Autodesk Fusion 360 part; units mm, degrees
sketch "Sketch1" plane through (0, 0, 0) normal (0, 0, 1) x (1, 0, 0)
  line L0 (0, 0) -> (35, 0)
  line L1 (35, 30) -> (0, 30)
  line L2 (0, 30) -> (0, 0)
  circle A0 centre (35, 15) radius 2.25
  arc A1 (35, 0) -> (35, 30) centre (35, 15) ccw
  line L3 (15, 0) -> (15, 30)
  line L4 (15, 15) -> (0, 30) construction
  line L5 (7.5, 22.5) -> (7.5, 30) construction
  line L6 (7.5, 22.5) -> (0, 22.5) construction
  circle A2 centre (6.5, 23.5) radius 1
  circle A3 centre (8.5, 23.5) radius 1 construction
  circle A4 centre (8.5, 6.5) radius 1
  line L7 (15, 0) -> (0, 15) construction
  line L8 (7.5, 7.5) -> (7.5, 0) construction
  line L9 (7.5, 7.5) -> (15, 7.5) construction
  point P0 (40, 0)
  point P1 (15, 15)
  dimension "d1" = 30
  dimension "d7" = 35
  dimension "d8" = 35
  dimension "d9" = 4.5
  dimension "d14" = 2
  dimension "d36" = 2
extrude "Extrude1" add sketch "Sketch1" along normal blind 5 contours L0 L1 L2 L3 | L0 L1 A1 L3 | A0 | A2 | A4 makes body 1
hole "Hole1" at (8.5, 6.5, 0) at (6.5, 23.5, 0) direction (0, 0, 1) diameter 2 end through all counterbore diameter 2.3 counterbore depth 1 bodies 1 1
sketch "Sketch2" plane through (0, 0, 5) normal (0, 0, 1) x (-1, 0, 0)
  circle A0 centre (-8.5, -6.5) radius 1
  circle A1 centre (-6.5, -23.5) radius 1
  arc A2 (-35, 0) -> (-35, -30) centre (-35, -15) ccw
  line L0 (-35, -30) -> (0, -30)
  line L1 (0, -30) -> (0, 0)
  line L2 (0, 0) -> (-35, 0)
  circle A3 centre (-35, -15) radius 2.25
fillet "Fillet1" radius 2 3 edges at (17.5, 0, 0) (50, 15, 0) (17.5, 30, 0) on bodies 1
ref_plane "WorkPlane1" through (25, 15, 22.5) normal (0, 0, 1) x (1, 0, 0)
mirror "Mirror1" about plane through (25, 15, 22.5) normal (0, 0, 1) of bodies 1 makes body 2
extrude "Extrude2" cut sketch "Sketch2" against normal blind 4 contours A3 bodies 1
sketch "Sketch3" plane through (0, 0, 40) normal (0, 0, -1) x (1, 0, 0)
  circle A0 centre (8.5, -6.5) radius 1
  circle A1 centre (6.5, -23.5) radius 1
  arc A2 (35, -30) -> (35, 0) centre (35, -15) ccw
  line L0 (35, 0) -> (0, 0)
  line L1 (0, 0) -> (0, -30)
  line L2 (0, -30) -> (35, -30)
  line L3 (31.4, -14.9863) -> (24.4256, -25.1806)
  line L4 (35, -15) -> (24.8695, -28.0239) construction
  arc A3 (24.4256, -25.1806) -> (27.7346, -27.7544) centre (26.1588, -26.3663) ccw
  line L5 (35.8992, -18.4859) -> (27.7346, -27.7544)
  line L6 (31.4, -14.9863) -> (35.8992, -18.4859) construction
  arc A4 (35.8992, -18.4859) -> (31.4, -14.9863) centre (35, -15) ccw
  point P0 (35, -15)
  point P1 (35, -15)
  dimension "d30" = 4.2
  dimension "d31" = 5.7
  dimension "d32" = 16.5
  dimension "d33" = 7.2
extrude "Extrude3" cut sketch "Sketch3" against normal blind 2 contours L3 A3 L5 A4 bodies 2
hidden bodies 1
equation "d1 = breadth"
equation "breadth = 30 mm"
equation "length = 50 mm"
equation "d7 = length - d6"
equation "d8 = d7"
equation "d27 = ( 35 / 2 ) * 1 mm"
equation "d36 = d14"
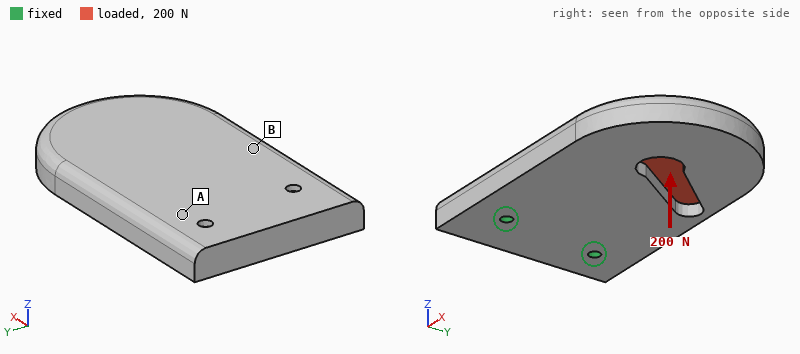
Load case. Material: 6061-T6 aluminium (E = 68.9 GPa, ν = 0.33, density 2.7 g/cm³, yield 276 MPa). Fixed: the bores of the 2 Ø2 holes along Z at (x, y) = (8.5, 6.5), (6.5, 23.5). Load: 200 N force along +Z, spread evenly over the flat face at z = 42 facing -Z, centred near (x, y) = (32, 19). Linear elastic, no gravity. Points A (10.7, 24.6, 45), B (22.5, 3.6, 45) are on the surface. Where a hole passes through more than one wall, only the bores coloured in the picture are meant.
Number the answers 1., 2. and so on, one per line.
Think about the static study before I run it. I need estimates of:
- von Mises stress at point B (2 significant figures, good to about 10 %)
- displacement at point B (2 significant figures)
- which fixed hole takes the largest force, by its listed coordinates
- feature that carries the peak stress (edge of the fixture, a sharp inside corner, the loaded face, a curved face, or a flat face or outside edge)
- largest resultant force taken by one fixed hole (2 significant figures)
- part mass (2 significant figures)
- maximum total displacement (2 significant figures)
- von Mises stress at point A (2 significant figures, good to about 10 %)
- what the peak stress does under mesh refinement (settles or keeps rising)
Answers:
1. 17 MPa
2. 0.028 mm
3. (6.5, 23.5)
4. edge of the fixture
5. 120 N
6. 18 g
7. 0.14 mm
8. 35 MPa
9. keeps rising
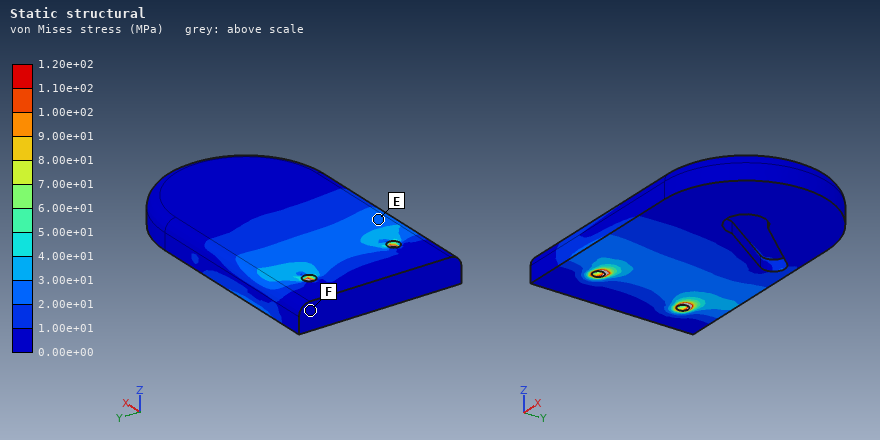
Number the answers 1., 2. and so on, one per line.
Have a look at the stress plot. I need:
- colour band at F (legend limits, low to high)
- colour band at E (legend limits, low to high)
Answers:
1. 0.00e+00 to 1.00e+01 MPa
2. 2.00e+01 to 3.00e+01 MPa
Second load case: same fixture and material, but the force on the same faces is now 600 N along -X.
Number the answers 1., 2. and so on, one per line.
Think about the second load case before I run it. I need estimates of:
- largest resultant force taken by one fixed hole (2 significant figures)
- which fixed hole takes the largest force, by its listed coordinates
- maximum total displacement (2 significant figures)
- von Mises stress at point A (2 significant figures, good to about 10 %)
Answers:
1. 450 N
2. (6.5, 23.5)
3. 15 µm
4. 7.0 MPa
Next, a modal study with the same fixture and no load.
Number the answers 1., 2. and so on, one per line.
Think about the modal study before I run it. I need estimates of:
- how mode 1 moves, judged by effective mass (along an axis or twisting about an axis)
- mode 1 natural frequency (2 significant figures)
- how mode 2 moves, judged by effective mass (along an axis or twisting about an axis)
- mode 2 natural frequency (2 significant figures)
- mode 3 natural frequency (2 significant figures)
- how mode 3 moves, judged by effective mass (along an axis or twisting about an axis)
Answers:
1. along Z
2. 2200 Hz
3. twisting about X
4. 7500 Hz
5. 9700 Hz
6. along Y
